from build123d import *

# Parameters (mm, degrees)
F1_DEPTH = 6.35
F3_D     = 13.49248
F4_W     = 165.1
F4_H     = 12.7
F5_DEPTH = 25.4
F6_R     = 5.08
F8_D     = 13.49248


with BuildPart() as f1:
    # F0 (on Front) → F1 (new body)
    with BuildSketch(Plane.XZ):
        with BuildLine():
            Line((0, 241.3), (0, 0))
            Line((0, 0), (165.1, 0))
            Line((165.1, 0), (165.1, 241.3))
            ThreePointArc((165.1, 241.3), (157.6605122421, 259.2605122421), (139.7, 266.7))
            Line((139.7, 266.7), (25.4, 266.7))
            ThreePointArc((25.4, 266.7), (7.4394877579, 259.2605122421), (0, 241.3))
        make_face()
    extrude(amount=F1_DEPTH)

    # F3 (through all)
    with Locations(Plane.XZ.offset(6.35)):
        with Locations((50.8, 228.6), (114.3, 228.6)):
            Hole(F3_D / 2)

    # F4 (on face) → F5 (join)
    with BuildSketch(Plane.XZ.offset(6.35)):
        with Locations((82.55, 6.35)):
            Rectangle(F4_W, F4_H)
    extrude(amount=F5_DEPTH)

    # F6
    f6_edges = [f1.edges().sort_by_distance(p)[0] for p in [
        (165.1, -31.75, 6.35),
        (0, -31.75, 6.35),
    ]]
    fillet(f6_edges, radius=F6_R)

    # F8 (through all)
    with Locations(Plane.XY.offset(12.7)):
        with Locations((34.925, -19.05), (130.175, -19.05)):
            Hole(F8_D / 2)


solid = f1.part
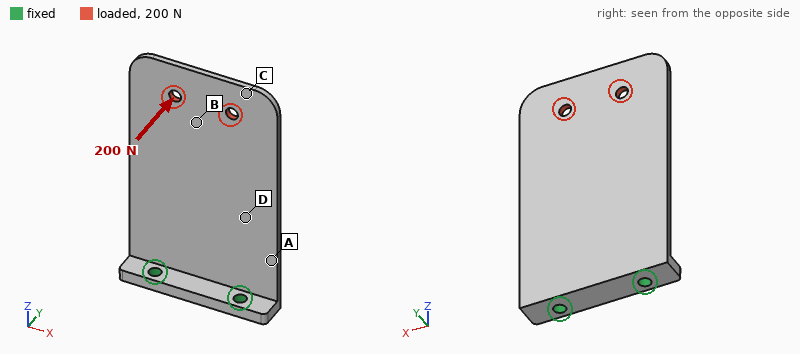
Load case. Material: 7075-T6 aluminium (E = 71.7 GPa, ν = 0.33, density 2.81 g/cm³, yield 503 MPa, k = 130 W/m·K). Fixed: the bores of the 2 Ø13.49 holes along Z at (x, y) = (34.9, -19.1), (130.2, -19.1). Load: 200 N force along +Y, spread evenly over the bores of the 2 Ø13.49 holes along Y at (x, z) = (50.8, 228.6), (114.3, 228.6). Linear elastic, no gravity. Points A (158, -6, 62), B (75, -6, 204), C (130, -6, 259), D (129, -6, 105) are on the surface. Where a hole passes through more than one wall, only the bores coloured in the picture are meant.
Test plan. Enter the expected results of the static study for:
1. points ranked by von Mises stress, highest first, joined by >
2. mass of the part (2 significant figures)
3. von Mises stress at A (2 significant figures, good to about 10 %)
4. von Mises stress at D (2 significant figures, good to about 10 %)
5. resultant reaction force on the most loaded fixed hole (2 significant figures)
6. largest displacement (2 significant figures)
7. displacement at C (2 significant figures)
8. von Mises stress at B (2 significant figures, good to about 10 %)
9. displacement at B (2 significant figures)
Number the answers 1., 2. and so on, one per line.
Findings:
1. A > D > B > C
2. 910 g
3. 30 MPa
4. 21 MPa
5. 120 N
6. 3.4 mm
7. 3.3 mm
8. 5.6 MPa
9. 2.3 mm
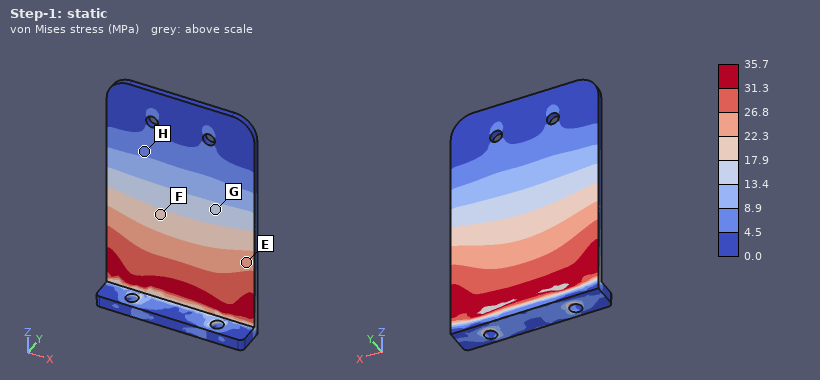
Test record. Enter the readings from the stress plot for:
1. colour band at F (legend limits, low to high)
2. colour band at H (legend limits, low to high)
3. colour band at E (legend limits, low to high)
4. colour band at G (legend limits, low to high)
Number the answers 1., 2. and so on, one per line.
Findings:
1. 17.9 to 22.3 MPa
2. 4.5 to 8.9 MPa
3. 22.3 to 26.8 MPa
4. 13.4 to 17.9 MPa
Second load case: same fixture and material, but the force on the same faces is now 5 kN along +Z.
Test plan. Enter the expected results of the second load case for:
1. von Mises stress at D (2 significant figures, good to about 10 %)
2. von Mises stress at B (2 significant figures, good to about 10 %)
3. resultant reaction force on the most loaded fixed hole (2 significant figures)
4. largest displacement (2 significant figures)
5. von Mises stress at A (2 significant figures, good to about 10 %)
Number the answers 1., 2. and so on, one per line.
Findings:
1. 4.8 MPa
2. 5.2 MPa
3. 2.5 kN
4. 0.13 mm
5. 4.6 MPa
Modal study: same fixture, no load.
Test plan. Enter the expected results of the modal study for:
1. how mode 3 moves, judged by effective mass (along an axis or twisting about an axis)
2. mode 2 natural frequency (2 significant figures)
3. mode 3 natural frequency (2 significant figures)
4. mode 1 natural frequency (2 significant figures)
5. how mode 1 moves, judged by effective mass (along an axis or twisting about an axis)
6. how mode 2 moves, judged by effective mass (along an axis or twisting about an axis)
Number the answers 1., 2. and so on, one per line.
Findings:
1. along Y
2. 280 Hz
3. 500 Hz
4. 81 Hz
5. along Y
6. twisting about Z
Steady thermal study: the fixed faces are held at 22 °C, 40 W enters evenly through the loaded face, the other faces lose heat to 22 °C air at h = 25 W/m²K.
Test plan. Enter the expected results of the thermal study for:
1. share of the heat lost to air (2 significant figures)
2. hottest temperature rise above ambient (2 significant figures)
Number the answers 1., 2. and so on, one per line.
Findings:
1. 76 %
2. 32 K
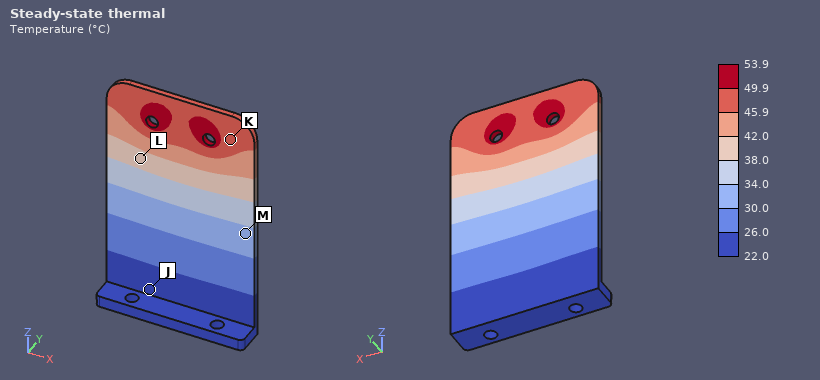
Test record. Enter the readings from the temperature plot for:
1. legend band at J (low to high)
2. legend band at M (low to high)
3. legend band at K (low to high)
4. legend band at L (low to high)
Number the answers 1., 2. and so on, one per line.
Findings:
1. 22.0 to 26.0 °C
2. 30.0 to 34.0 °C
3. 45.9 to 49.9 °C
4. 38.0 to 42.0 °C
